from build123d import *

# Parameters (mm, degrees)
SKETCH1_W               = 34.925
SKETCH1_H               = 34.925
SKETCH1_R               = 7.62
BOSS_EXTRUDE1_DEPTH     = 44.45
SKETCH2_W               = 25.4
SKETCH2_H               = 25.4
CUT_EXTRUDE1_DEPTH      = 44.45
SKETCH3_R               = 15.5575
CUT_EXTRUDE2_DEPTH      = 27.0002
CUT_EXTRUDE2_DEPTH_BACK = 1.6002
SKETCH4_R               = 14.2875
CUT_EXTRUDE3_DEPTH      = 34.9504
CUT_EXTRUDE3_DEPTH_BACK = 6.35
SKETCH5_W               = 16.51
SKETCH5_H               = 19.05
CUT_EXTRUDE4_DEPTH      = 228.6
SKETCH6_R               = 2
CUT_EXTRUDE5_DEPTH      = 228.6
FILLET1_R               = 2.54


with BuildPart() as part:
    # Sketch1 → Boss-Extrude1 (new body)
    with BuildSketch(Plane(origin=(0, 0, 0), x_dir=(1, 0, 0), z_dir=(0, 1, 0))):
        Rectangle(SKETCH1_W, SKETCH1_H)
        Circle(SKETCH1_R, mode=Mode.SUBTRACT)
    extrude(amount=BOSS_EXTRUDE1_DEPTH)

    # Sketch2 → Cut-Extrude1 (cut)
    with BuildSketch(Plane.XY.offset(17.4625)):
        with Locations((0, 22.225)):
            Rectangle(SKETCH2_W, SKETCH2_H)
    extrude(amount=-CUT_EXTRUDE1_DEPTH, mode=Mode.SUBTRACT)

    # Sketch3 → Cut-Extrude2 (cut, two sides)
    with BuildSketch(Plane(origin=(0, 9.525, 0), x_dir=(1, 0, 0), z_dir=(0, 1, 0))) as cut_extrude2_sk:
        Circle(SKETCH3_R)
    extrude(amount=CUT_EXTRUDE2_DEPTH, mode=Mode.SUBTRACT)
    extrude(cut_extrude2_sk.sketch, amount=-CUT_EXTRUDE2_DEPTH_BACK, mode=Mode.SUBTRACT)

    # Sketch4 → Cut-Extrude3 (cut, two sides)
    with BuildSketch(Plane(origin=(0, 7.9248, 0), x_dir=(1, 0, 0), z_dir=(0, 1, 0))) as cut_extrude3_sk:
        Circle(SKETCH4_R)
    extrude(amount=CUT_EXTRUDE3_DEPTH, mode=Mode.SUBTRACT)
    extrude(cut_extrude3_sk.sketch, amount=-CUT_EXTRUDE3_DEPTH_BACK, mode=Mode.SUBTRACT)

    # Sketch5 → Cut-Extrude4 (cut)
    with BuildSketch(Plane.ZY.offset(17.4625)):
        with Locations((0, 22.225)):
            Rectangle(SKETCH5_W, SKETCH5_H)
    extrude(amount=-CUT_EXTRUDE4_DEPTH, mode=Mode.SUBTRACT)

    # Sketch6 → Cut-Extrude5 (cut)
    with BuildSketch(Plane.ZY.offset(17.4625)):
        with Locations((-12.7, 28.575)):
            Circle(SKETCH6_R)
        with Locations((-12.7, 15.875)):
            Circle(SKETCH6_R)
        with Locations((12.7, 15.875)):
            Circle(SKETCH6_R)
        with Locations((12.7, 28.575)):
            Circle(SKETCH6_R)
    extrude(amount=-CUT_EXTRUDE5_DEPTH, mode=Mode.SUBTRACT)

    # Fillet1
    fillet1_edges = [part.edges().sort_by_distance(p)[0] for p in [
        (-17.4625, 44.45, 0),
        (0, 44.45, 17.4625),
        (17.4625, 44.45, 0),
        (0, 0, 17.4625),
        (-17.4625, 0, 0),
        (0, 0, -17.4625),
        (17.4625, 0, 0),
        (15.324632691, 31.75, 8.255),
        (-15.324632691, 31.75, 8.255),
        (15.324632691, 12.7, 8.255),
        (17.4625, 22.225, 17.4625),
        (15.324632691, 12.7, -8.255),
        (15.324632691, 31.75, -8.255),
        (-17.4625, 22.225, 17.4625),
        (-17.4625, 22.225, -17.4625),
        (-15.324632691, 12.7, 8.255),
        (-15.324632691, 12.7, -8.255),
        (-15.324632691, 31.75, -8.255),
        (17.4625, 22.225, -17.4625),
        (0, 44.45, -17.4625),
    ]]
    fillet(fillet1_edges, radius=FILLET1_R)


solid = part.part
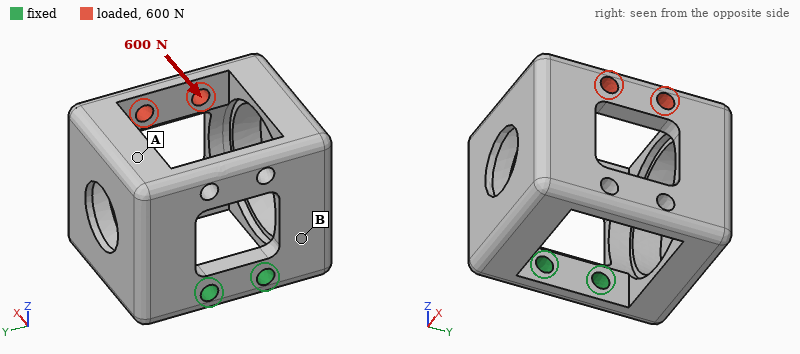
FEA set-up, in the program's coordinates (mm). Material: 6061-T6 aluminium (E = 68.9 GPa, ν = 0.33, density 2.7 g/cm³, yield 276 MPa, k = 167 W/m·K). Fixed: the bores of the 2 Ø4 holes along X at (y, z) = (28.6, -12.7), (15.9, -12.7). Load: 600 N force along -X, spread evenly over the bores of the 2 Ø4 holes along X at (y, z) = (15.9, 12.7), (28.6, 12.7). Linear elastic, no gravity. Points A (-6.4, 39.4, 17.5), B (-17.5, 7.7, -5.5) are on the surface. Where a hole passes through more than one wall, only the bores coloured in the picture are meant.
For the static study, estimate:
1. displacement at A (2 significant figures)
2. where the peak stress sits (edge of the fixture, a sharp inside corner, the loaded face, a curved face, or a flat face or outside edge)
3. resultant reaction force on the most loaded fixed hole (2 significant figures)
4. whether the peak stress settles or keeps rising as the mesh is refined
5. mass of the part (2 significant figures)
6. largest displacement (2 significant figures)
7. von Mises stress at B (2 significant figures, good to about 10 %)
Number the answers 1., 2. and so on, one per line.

1. 0.29 mm
2. edge of the fixture
3. 310 N
4. keeps rising
5. 43 g
6. 0.40 mm
7. 70 MPa
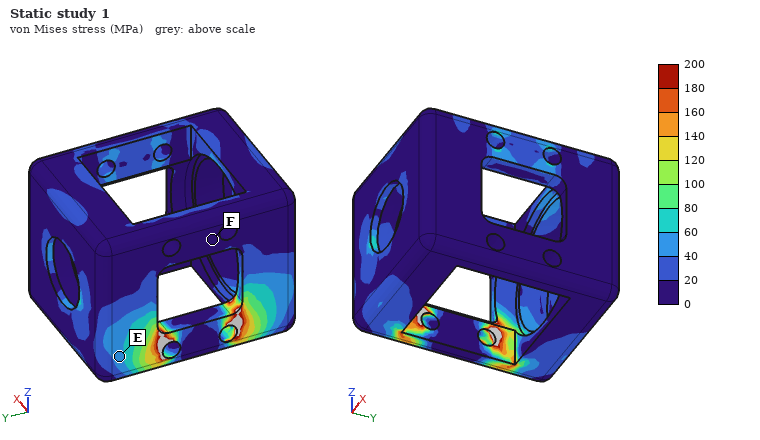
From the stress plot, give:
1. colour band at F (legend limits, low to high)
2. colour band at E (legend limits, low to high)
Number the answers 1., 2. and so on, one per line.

1. 0 to 20 MPa
2. 40 to 60 MPa
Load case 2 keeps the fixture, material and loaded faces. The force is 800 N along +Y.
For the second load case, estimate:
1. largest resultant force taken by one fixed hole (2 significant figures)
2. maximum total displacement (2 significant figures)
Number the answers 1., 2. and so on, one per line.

1. 1.1 kN
2. 0.31 mm
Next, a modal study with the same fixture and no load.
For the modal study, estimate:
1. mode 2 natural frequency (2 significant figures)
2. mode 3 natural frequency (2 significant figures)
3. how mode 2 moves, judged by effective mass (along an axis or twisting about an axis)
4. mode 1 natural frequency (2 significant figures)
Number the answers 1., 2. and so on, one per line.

1. 1800 Hz
2. 3200 Hz
3. along Y
4. 1200 Hz
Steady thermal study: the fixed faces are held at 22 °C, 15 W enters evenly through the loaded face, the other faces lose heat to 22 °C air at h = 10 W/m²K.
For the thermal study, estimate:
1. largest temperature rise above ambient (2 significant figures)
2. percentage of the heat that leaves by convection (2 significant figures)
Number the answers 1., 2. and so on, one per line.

1. 35 K
2. 11 %
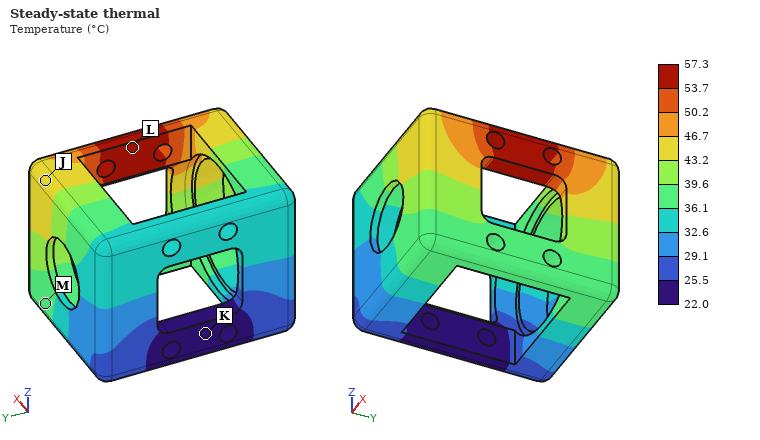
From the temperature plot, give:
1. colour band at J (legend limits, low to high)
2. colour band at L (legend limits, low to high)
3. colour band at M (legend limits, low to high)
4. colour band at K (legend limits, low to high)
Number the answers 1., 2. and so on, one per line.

1. 43.2 to 46.7 °C
2. 53.7 to 57.3 °C
3. 36.1 to 39.6 °C
4. 22.0 to 25.5 °C
